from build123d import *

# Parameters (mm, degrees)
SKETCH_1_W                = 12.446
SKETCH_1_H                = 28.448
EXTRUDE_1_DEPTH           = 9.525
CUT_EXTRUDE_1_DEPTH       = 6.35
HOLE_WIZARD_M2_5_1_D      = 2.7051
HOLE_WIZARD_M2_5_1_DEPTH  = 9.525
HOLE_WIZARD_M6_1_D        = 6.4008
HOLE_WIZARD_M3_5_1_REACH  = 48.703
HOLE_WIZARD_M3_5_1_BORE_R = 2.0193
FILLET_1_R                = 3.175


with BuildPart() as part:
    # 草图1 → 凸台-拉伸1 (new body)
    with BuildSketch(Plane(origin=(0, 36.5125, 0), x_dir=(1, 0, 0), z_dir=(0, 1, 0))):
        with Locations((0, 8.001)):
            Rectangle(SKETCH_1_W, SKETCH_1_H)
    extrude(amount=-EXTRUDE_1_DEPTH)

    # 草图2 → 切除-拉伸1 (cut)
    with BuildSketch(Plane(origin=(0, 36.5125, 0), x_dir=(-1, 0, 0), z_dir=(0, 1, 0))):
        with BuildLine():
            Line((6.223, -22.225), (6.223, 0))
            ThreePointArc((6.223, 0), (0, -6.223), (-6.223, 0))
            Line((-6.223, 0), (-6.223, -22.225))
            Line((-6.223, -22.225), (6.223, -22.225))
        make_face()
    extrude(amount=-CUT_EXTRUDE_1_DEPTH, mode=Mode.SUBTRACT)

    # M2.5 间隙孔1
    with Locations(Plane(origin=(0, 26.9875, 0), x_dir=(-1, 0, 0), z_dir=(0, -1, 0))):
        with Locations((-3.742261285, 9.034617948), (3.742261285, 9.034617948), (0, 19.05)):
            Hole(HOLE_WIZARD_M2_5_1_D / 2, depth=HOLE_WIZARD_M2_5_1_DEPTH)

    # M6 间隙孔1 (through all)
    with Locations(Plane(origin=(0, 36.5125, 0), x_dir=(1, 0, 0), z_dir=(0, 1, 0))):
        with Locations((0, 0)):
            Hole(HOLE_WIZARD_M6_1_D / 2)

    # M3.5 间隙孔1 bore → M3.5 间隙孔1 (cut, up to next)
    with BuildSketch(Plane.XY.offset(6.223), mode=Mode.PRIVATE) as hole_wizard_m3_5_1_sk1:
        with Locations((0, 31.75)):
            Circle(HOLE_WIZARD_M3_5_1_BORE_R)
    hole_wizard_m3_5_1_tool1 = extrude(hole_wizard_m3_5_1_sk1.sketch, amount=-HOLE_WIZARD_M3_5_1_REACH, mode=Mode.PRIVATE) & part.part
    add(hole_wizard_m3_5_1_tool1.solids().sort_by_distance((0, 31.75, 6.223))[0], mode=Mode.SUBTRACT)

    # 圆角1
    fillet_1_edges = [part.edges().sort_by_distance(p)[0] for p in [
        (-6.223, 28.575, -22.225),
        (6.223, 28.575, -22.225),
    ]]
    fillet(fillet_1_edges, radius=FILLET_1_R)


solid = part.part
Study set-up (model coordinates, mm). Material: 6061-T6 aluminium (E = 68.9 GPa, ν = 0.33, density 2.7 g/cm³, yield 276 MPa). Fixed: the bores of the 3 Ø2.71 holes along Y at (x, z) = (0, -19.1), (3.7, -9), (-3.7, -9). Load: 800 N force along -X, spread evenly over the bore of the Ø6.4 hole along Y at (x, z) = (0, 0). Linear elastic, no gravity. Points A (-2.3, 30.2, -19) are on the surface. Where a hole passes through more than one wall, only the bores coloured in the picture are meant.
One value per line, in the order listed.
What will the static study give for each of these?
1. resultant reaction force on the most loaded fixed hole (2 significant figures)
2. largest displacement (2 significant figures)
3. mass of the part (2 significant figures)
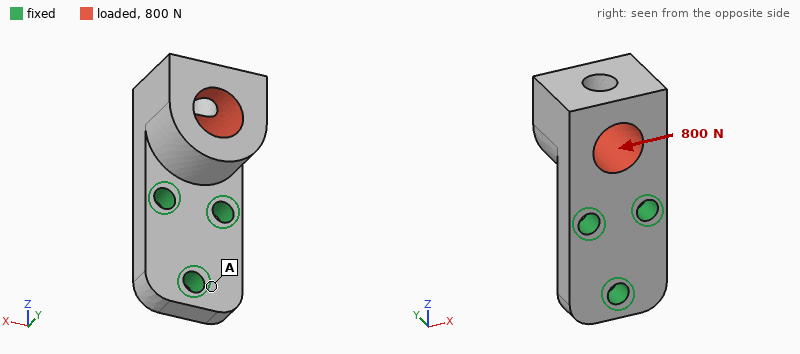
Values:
870 N
33 µm
4.3 g
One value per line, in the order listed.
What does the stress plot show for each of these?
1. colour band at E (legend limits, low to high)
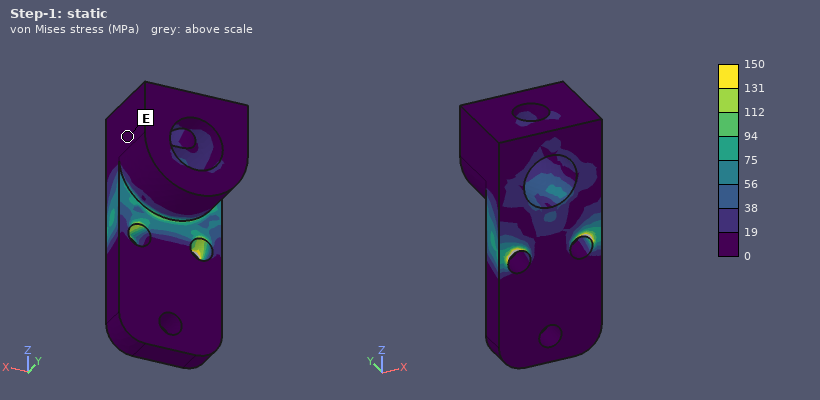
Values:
0 to 19 MPa
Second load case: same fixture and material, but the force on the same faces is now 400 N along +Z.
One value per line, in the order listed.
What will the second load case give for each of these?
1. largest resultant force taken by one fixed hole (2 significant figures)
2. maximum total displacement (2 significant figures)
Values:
200 N
37 µm
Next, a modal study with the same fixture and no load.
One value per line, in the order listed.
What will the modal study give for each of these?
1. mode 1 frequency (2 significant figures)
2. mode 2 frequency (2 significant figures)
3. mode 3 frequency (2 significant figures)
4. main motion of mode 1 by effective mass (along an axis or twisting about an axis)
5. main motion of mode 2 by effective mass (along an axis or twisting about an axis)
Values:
7700 Hz
18 kHz
22 kHz
along Y
along X
